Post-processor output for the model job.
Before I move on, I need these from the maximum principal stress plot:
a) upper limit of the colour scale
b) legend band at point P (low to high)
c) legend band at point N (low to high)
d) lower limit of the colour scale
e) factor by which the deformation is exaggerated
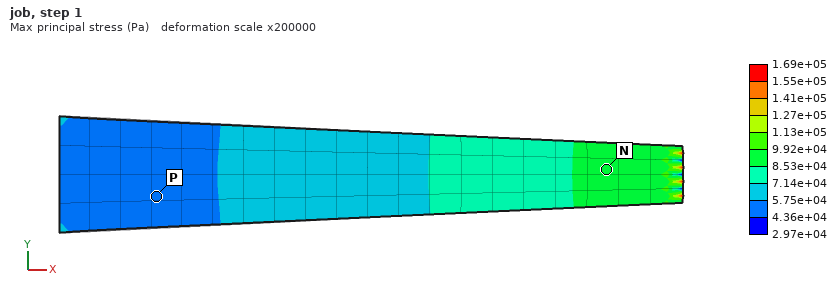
1.69e+05 Pa
4.36e+04 to 5.75e+04 Pa
8.53e+04 to 9.92e+04 Pa
2.97e+04 Pa
200000
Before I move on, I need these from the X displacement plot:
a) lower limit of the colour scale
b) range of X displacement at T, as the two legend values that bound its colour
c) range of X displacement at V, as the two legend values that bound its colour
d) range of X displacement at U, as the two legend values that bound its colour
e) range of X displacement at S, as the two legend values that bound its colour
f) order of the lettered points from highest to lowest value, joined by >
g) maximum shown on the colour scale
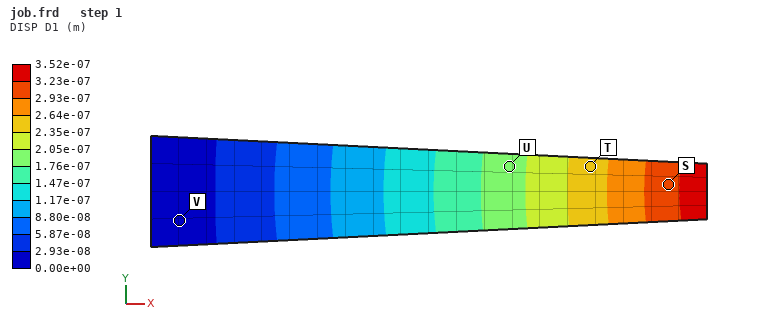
0.00e+00 m
2.35e-07 to 2.64e-07 m
0.00e+00 to 2.93e-08 m
1.76e-07 to 2.05e-07 m
2.93e-07 to 3.23e-07 m
S > T > U > V
3.52e-07 m
